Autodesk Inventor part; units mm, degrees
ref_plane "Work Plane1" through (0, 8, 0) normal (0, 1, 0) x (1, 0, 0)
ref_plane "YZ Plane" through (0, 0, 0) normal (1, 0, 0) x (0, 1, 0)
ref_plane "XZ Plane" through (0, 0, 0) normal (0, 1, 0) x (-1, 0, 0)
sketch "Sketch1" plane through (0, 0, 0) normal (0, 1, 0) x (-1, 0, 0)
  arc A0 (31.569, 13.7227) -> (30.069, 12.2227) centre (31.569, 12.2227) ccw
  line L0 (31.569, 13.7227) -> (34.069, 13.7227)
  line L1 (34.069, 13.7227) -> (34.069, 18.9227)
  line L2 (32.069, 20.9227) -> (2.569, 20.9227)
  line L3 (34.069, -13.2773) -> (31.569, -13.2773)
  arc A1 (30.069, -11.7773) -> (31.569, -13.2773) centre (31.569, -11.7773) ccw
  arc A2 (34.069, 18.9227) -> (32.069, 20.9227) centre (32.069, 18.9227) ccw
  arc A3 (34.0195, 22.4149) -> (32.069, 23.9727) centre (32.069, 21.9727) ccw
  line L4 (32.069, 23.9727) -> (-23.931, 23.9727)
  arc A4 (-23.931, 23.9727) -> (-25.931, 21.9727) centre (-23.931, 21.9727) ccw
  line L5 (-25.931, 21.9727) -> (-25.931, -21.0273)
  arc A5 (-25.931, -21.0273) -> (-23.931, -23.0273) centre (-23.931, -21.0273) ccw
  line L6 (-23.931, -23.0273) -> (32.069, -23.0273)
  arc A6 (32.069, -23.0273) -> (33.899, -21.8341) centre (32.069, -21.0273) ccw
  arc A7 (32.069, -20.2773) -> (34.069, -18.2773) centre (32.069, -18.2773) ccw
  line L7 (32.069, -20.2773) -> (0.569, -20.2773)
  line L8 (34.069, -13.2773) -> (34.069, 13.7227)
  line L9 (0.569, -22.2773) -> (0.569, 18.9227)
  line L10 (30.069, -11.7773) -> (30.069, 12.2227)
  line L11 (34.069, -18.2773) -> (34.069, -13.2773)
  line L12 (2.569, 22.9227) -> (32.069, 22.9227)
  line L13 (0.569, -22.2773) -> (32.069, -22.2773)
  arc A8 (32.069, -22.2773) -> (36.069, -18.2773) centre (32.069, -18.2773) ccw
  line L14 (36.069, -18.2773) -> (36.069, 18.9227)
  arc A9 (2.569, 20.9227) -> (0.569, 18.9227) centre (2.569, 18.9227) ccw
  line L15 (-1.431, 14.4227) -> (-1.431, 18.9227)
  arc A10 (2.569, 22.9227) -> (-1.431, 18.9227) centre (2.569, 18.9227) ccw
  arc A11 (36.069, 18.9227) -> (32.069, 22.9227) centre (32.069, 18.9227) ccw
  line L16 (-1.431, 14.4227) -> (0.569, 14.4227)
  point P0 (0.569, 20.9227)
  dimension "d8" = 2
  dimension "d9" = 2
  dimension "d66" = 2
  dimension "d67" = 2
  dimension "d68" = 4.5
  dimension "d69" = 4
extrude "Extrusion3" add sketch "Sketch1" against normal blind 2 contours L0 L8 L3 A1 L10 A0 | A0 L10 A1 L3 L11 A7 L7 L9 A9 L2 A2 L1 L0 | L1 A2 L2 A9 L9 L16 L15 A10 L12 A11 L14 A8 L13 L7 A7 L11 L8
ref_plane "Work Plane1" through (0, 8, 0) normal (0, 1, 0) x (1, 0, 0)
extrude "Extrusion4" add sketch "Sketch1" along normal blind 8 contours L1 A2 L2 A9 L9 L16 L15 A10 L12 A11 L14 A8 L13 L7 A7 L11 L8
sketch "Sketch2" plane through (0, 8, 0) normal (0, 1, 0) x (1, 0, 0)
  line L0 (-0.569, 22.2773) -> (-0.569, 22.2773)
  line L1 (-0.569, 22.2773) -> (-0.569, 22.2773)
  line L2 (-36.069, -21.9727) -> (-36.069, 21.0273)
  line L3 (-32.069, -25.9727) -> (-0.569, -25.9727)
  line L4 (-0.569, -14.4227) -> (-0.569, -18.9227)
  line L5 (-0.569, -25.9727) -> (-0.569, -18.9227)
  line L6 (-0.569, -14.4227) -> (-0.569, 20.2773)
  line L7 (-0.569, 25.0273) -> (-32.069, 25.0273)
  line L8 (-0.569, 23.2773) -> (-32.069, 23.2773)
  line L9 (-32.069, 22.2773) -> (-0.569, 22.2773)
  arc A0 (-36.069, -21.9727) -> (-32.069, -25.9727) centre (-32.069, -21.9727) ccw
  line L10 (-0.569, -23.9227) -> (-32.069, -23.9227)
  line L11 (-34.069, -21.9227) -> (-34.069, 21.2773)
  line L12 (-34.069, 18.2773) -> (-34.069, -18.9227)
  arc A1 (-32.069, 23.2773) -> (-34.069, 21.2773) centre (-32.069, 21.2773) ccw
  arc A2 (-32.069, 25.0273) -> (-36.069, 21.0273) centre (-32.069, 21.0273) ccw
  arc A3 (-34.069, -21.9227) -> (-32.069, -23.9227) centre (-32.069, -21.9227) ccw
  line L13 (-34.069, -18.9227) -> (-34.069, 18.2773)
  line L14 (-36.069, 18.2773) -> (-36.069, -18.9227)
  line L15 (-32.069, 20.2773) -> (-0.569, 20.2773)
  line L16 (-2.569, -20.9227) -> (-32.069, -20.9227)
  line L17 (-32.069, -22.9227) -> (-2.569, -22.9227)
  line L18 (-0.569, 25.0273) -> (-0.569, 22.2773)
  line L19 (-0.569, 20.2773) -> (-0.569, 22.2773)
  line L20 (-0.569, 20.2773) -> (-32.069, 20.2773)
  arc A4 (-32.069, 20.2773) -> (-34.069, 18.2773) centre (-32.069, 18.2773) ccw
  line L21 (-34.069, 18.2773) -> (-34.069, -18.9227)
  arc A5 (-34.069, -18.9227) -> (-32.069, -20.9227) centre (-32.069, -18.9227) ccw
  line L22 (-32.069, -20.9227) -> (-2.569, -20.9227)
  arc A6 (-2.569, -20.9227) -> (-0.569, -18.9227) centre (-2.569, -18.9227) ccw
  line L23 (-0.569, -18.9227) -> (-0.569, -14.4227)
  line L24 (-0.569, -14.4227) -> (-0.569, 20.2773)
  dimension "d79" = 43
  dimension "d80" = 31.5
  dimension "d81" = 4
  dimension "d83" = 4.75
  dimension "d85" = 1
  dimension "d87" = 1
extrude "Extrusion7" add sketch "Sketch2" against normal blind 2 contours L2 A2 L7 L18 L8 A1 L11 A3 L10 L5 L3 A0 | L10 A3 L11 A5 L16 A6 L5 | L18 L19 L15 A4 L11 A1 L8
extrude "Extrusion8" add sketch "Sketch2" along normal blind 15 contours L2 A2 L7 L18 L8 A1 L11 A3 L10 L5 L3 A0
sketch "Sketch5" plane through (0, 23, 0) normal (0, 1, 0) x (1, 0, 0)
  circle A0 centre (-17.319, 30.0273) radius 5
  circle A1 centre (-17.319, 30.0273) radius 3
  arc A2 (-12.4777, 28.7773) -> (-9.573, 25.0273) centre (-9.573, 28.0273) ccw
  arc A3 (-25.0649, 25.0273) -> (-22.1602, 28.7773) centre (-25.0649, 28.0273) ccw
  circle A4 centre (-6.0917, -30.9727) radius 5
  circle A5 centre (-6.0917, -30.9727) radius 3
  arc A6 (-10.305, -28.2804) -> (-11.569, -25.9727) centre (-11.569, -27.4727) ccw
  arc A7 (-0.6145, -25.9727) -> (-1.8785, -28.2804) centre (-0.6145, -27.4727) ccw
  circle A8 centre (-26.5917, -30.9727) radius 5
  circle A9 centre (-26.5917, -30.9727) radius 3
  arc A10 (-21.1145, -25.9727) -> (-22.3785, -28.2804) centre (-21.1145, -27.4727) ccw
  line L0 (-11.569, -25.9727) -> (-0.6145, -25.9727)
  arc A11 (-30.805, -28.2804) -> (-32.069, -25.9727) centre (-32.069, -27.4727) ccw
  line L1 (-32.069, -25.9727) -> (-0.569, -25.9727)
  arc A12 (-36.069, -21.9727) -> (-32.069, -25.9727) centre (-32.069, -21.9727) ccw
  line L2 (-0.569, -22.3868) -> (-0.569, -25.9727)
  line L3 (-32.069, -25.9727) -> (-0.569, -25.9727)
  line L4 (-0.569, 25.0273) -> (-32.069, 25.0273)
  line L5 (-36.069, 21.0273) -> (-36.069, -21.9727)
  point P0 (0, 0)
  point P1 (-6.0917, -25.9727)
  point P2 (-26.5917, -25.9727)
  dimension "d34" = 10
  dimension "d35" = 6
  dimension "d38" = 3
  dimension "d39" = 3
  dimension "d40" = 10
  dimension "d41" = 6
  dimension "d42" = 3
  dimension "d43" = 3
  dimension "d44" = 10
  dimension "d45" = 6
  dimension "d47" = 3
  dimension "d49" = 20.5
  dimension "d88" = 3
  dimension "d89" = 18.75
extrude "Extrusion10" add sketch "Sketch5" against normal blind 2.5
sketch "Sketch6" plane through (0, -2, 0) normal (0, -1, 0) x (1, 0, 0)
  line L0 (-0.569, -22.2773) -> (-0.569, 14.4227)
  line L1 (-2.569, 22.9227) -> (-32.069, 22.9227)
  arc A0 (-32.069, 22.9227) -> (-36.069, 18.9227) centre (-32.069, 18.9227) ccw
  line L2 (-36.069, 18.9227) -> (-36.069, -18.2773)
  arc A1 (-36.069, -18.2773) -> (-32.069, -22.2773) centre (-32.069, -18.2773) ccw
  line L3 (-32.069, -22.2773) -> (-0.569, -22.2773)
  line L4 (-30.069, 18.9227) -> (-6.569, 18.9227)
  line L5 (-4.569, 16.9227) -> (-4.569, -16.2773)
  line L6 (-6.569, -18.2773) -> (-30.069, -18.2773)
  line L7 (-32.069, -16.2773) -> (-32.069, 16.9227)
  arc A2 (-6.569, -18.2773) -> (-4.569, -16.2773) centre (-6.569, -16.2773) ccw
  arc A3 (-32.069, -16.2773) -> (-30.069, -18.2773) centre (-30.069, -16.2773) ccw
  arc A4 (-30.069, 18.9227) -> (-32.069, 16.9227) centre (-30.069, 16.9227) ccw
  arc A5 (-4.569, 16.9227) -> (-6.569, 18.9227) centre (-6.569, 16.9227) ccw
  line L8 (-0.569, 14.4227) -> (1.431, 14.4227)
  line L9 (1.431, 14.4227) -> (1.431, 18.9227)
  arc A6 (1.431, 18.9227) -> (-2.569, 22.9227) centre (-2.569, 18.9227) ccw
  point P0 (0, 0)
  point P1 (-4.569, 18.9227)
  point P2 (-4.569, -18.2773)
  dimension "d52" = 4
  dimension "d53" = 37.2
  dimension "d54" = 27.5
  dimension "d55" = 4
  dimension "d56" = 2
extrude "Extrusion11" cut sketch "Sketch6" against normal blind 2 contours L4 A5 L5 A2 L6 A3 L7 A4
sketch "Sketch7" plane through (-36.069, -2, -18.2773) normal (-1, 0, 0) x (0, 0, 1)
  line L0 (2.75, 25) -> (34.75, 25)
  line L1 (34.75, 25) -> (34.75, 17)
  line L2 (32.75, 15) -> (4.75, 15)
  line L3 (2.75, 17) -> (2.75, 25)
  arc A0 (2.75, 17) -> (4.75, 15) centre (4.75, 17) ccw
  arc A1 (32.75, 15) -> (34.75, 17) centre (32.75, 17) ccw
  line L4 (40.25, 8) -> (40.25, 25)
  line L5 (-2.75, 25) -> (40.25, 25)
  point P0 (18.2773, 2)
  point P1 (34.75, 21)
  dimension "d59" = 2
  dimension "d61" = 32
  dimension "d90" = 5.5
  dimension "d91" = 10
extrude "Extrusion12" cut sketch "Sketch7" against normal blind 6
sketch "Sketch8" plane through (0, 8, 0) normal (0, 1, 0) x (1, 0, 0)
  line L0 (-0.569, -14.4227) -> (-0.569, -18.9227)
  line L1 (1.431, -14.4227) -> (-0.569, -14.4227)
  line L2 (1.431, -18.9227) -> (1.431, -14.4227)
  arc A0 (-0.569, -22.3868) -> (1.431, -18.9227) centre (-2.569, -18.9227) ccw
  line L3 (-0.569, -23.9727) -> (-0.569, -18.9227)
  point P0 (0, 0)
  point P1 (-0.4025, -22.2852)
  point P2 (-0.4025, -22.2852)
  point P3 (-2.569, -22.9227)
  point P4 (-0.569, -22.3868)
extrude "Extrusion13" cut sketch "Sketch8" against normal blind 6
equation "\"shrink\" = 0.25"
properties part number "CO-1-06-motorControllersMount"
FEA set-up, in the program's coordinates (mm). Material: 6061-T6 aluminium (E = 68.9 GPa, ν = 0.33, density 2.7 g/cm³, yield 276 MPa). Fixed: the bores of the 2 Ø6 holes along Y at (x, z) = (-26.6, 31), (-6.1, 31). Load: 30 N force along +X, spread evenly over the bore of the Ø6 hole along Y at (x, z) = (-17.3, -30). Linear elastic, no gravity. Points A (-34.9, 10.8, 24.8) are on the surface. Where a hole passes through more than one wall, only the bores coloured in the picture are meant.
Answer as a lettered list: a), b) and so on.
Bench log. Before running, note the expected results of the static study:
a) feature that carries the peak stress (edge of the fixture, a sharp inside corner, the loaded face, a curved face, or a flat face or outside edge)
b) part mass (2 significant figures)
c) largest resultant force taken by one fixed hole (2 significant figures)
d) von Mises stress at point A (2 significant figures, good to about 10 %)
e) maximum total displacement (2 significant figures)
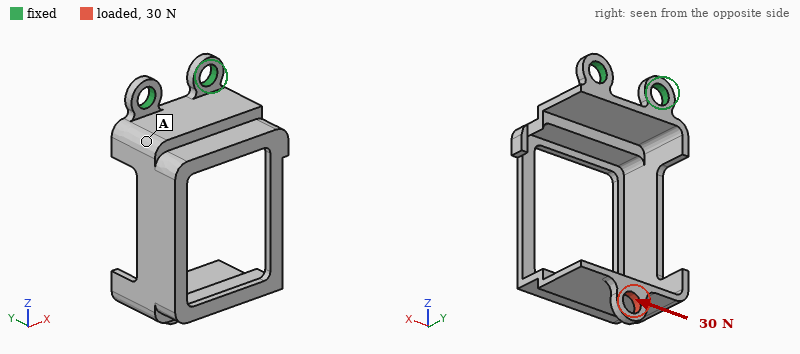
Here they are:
a) a curved face
b) 18 g
c) 61 N
d) 22 MPa
e) 0.82 mm
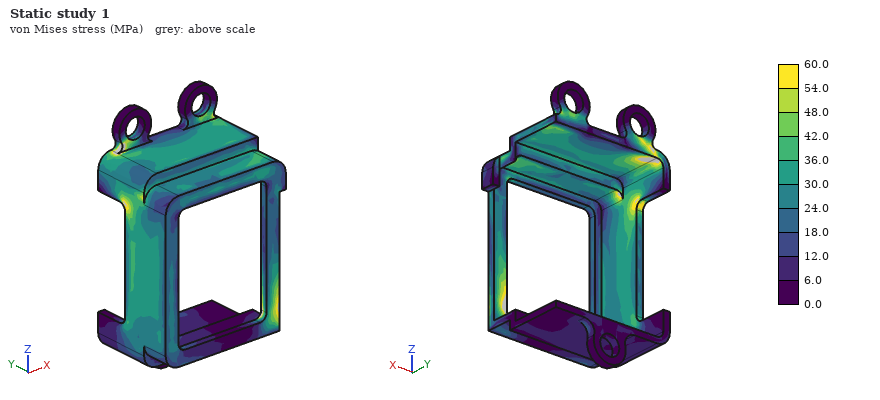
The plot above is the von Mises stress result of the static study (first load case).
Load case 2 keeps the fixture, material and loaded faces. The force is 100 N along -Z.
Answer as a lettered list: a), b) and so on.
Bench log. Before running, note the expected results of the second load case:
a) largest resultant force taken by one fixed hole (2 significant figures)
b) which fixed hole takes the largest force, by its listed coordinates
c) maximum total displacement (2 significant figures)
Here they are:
a) 61 N
b) (-6.1, 31)
c) 0.95 mm
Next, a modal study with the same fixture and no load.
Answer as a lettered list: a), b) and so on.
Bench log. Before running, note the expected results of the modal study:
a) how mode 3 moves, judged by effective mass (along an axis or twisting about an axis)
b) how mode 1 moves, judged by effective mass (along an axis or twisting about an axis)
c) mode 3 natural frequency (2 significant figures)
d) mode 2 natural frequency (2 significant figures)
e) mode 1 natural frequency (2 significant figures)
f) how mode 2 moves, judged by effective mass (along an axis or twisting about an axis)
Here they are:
a) along Z
b) along Y
c) 1200 Hz
d) 490 Hz
e) 370 Hz
f) along X
